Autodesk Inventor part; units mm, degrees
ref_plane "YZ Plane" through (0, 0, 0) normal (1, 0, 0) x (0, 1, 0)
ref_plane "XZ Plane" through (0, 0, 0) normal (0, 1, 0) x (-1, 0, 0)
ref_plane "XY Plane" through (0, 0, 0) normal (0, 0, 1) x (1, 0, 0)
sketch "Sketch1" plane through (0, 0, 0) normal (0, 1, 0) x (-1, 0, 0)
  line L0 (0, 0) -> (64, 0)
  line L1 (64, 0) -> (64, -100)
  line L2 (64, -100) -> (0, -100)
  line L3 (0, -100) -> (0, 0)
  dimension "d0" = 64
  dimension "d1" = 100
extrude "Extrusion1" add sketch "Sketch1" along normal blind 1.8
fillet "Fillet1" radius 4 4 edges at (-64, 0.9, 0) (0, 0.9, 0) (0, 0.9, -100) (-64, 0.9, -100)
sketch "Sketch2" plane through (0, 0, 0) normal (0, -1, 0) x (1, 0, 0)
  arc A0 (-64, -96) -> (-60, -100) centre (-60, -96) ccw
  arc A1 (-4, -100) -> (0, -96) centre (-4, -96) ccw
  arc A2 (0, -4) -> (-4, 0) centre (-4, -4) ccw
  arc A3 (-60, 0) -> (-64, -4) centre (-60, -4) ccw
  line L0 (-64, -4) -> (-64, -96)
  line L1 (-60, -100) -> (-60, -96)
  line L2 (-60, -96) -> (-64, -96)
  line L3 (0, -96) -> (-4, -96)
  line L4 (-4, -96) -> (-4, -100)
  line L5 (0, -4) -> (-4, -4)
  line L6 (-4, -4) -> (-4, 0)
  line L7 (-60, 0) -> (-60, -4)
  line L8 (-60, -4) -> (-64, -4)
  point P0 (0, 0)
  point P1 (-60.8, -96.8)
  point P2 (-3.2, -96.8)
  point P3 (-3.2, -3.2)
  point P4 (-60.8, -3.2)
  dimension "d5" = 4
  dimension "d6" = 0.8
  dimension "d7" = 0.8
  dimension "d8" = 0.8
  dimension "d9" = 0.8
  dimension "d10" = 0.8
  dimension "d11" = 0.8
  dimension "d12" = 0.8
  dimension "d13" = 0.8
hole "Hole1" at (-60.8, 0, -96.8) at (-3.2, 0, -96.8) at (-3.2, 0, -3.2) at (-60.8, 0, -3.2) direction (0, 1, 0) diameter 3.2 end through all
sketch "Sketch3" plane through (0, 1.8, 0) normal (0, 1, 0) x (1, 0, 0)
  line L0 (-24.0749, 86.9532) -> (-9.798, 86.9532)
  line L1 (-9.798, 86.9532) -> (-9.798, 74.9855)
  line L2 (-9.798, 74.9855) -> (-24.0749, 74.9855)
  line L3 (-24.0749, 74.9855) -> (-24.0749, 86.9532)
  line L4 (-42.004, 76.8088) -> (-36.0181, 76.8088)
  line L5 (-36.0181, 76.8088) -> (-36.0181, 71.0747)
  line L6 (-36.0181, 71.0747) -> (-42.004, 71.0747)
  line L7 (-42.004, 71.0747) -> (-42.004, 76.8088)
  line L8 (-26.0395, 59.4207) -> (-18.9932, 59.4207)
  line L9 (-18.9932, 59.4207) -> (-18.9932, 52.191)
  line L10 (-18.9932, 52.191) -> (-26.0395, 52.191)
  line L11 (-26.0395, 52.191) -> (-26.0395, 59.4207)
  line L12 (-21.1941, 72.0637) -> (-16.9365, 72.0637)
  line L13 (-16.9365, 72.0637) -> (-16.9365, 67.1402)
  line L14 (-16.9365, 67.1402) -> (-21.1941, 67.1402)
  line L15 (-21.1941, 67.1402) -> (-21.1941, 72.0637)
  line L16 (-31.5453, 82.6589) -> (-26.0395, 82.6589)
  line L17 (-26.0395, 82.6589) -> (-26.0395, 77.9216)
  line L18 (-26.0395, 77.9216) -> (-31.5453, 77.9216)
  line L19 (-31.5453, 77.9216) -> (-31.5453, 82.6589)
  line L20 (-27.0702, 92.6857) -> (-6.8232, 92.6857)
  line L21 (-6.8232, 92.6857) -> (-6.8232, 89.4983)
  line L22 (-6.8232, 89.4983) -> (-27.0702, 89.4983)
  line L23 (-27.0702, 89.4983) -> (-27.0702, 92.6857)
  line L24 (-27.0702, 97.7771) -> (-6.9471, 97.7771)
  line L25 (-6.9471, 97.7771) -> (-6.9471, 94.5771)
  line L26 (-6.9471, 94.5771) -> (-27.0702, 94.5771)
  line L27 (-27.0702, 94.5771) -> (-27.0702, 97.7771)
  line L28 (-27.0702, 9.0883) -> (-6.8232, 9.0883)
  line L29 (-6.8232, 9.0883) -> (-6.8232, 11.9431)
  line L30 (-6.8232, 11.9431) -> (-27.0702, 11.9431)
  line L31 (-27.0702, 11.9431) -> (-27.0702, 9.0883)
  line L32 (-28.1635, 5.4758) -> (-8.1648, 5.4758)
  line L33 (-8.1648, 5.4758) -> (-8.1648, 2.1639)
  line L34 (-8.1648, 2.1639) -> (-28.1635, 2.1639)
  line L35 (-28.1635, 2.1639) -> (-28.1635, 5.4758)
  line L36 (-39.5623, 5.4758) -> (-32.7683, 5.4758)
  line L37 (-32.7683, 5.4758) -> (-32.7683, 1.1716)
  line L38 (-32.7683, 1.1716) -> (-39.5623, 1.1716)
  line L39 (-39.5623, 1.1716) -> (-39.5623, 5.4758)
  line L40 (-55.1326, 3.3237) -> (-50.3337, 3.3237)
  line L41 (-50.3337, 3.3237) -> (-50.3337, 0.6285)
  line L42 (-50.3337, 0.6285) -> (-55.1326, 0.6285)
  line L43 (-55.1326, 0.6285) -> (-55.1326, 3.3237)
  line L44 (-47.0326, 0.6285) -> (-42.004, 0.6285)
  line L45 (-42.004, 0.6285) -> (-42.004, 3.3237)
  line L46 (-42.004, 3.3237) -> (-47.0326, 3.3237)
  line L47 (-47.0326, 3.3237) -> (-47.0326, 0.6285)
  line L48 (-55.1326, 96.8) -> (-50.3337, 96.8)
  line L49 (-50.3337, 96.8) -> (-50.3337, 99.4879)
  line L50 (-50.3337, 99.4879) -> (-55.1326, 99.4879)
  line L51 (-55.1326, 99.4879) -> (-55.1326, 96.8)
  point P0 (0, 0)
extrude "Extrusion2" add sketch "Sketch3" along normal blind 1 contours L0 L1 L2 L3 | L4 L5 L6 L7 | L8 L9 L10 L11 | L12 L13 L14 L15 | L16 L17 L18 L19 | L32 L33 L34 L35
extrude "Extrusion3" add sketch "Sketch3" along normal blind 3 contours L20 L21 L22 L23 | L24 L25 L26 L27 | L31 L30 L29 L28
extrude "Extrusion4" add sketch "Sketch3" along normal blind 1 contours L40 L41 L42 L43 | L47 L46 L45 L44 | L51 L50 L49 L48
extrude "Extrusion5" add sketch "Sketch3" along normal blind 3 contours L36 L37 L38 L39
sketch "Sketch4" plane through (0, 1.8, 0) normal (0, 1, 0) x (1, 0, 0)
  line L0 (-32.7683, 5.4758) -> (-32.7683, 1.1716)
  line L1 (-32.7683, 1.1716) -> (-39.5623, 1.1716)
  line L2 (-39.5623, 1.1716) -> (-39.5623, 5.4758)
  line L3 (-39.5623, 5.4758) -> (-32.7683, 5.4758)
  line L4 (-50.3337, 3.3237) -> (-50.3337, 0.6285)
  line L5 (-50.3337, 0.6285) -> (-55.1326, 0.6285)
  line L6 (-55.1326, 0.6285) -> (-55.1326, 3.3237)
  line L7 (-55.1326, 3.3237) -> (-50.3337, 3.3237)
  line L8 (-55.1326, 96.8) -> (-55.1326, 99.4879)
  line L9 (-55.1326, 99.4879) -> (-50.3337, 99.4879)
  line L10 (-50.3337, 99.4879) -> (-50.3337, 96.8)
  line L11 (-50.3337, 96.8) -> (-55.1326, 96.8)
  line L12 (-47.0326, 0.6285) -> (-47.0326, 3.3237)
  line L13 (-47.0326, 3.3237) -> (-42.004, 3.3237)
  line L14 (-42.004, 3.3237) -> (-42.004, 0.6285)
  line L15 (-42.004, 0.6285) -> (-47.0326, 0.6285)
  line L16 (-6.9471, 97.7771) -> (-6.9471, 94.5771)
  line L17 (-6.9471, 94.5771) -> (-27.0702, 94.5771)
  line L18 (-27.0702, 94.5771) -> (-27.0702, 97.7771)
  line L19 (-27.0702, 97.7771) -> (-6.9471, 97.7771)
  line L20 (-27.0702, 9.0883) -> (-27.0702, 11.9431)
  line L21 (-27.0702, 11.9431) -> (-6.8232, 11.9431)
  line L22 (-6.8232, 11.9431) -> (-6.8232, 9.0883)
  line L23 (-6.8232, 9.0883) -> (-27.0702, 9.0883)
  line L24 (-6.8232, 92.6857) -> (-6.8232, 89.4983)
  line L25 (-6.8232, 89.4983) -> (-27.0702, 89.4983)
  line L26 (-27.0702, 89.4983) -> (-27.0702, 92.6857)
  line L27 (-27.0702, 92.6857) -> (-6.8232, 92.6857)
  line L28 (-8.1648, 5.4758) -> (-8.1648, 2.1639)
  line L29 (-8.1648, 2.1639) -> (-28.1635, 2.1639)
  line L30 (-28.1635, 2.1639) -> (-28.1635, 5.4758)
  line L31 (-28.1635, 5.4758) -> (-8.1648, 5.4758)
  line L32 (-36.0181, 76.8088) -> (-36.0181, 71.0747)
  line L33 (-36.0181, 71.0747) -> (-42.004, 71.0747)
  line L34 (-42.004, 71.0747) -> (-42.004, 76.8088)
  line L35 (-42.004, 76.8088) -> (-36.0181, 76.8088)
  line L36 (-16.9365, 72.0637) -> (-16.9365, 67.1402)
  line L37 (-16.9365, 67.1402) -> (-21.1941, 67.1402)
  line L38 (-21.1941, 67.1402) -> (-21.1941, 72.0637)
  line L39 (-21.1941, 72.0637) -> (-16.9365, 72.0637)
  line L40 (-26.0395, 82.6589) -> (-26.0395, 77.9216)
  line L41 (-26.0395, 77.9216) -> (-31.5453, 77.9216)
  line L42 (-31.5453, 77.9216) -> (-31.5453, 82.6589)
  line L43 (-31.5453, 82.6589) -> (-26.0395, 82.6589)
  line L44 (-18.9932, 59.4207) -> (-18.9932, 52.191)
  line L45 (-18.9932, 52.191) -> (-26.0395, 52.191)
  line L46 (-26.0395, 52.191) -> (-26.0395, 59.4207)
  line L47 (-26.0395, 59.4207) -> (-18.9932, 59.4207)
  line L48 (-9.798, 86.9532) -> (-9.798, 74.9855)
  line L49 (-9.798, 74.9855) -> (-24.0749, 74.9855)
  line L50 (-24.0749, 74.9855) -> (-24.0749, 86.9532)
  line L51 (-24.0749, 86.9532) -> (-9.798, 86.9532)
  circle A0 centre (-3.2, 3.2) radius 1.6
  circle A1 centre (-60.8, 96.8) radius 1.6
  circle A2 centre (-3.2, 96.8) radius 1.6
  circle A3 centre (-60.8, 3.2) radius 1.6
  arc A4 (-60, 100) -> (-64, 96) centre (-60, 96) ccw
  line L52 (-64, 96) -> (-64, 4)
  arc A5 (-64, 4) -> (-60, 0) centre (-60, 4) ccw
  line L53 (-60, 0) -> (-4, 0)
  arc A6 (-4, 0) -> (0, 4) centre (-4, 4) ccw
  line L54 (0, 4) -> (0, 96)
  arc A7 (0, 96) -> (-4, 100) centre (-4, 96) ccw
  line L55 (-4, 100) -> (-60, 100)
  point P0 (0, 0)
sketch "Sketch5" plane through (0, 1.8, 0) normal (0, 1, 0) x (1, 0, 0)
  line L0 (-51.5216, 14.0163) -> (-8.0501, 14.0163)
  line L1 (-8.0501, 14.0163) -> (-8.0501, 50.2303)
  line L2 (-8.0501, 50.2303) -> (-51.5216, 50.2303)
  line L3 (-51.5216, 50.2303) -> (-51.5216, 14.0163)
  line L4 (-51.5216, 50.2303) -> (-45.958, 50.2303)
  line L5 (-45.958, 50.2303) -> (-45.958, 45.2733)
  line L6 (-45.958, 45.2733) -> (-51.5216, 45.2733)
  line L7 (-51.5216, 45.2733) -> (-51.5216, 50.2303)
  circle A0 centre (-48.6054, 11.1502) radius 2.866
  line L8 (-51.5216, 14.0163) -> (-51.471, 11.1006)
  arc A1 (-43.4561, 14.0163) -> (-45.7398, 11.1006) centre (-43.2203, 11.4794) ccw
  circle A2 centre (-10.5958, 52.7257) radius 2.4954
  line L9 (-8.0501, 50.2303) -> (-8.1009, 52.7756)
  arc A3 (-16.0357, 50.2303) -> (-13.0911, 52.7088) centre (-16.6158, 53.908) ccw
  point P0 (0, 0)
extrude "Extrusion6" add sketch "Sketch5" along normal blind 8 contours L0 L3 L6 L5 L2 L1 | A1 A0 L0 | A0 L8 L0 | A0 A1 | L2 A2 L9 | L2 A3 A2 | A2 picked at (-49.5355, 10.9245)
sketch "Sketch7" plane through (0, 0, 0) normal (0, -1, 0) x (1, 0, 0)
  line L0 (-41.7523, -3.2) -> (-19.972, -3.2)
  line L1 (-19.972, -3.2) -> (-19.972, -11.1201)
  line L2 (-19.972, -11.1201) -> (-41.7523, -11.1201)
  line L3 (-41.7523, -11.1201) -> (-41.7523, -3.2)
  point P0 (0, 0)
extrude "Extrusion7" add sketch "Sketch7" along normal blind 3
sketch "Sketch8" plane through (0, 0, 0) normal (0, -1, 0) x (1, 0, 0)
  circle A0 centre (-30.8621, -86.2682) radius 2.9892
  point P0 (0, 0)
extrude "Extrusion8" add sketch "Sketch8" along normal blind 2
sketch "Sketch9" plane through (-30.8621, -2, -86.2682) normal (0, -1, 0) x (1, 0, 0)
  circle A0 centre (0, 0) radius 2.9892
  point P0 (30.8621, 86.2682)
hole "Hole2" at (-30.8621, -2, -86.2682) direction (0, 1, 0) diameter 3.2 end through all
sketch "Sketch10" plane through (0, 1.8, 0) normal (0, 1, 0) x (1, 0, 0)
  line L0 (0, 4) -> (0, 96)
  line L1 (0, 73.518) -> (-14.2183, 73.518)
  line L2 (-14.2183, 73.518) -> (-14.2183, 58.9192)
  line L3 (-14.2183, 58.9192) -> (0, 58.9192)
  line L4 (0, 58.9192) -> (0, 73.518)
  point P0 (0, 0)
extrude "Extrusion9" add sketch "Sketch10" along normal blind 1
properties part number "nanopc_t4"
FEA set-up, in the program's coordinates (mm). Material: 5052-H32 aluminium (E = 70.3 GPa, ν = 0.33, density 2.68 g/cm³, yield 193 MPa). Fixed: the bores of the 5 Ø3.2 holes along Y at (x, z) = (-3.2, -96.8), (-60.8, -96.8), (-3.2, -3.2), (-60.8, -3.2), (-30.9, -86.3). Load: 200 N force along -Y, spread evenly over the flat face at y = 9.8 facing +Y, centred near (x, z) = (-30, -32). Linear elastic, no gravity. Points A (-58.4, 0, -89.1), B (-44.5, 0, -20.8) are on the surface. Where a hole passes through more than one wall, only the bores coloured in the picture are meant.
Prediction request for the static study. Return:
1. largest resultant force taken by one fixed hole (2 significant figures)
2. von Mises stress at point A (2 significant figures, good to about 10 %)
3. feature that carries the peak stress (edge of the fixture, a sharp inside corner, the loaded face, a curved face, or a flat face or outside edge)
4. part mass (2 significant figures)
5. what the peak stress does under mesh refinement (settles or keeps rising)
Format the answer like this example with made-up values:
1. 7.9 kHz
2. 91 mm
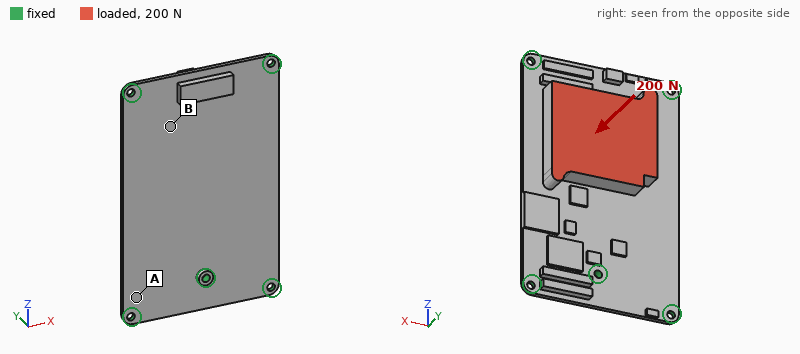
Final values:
1. 92 N
2. 12 MPa
3. edge of the fixture
4. 70 g
5. keeps rising
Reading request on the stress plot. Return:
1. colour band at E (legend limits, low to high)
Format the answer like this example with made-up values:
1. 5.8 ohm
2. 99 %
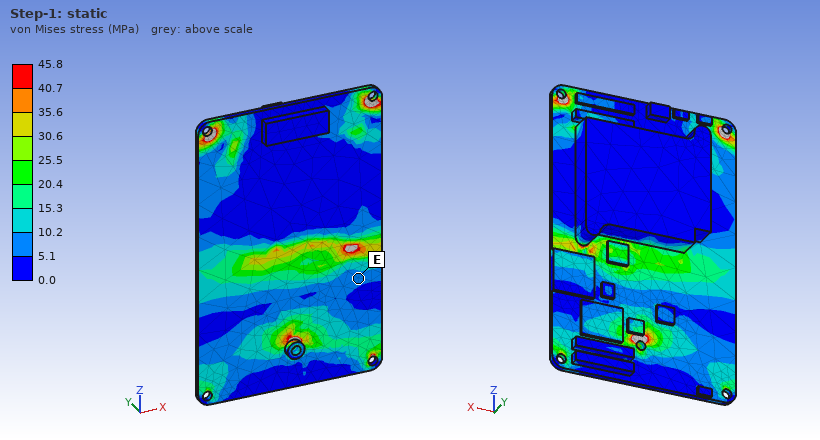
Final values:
1. 5.1 to 10.2 MPa
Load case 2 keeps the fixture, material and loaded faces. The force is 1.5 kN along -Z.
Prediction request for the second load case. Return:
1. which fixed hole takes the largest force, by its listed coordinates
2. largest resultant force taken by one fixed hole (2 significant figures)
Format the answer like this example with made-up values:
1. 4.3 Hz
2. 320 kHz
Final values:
1. (-30.9, -86.3)
2. 480 N
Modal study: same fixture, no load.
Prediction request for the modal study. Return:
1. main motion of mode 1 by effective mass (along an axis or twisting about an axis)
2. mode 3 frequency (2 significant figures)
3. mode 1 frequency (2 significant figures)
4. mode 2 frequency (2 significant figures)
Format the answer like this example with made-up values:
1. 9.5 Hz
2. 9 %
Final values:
1. along Y
2. 3200 Hz
3. 1100 Hz
4. 2500 Hz
